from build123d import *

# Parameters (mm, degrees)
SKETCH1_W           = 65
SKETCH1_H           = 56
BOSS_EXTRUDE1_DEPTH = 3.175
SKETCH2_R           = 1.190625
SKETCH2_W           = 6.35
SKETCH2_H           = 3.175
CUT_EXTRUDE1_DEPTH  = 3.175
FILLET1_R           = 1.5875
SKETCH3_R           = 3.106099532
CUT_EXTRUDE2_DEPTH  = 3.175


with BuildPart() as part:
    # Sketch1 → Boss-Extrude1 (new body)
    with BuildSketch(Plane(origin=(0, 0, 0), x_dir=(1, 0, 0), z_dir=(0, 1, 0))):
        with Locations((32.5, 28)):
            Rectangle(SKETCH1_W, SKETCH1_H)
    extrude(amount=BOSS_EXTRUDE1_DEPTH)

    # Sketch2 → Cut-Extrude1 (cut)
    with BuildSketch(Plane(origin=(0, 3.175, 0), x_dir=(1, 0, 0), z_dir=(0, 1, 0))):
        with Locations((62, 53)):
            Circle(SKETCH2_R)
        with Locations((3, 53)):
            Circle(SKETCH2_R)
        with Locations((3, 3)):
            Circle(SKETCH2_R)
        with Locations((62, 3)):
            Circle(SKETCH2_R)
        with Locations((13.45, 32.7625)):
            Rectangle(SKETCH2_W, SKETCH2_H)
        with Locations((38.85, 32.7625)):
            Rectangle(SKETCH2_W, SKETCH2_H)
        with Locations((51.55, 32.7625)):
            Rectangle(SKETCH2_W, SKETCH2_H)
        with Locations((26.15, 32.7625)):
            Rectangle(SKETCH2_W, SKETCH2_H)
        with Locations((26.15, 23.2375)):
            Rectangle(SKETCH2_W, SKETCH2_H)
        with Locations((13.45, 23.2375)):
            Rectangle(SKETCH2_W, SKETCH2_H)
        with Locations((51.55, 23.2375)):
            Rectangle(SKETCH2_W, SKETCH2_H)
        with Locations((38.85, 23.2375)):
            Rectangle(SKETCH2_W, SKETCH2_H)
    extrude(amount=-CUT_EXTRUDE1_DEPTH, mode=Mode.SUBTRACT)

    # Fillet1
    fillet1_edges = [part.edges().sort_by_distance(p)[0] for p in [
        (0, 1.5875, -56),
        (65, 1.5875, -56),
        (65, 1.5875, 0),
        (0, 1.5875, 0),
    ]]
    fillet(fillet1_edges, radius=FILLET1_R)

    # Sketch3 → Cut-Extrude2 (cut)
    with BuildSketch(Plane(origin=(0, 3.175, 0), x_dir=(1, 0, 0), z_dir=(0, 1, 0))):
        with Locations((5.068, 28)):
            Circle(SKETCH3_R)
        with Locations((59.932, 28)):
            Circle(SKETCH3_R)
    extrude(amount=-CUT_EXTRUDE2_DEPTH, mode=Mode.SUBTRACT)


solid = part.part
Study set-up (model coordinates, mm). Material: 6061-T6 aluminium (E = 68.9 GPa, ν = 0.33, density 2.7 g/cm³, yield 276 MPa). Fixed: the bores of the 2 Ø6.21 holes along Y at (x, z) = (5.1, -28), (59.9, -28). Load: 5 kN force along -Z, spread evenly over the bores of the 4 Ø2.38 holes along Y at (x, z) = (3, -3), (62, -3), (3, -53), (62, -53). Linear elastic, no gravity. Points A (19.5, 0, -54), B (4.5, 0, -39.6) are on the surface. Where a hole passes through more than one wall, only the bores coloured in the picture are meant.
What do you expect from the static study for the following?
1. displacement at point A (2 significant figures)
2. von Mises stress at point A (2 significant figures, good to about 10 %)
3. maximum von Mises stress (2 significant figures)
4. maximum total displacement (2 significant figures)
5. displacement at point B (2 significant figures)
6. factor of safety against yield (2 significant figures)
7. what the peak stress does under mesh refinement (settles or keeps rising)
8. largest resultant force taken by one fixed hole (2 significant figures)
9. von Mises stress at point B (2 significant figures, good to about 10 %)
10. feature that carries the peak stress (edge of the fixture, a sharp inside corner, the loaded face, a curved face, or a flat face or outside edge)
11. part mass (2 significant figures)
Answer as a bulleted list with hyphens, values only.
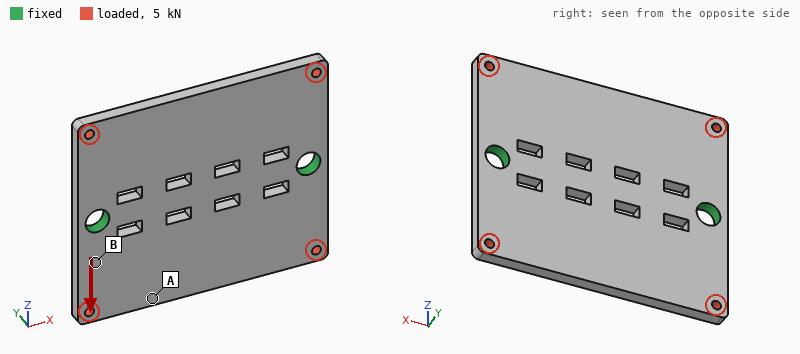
- 4.2 µm
- 11 MPa
- 160 MPa
- 20 µm
- 5.4 µm
- 1.8
- settles
- 2.5 kN
- 39 MPa
- the loaded face
- 29 g
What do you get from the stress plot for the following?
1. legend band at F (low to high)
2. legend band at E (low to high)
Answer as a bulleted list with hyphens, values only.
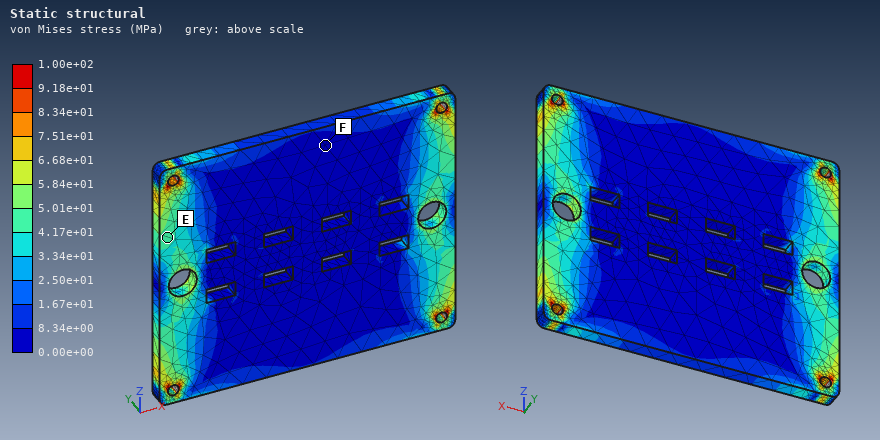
- 0.00e+00 to 8.34e+00 MPa
- 4.17e+01 to 5.01e+01 MPa
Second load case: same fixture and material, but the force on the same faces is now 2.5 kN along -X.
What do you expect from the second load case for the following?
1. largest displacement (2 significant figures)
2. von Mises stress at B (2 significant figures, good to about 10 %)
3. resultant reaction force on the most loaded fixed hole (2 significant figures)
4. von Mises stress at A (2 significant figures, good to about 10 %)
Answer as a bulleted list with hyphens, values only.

- 18 µm
- 9.3 MPa
- 1.3 kN
- 14 MPa
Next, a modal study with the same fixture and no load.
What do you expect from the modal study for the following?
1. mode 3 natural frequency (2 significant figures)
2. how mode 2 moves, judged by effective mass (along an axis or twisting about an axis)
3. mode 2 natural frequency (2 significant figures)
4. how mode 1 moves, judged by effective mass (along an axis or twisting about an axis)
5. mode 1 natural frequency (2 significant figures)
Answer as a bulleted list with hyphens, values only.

- 4900 Hz
- along Y
- 2800 Hz
- twisting about X
- 2300 Hz
